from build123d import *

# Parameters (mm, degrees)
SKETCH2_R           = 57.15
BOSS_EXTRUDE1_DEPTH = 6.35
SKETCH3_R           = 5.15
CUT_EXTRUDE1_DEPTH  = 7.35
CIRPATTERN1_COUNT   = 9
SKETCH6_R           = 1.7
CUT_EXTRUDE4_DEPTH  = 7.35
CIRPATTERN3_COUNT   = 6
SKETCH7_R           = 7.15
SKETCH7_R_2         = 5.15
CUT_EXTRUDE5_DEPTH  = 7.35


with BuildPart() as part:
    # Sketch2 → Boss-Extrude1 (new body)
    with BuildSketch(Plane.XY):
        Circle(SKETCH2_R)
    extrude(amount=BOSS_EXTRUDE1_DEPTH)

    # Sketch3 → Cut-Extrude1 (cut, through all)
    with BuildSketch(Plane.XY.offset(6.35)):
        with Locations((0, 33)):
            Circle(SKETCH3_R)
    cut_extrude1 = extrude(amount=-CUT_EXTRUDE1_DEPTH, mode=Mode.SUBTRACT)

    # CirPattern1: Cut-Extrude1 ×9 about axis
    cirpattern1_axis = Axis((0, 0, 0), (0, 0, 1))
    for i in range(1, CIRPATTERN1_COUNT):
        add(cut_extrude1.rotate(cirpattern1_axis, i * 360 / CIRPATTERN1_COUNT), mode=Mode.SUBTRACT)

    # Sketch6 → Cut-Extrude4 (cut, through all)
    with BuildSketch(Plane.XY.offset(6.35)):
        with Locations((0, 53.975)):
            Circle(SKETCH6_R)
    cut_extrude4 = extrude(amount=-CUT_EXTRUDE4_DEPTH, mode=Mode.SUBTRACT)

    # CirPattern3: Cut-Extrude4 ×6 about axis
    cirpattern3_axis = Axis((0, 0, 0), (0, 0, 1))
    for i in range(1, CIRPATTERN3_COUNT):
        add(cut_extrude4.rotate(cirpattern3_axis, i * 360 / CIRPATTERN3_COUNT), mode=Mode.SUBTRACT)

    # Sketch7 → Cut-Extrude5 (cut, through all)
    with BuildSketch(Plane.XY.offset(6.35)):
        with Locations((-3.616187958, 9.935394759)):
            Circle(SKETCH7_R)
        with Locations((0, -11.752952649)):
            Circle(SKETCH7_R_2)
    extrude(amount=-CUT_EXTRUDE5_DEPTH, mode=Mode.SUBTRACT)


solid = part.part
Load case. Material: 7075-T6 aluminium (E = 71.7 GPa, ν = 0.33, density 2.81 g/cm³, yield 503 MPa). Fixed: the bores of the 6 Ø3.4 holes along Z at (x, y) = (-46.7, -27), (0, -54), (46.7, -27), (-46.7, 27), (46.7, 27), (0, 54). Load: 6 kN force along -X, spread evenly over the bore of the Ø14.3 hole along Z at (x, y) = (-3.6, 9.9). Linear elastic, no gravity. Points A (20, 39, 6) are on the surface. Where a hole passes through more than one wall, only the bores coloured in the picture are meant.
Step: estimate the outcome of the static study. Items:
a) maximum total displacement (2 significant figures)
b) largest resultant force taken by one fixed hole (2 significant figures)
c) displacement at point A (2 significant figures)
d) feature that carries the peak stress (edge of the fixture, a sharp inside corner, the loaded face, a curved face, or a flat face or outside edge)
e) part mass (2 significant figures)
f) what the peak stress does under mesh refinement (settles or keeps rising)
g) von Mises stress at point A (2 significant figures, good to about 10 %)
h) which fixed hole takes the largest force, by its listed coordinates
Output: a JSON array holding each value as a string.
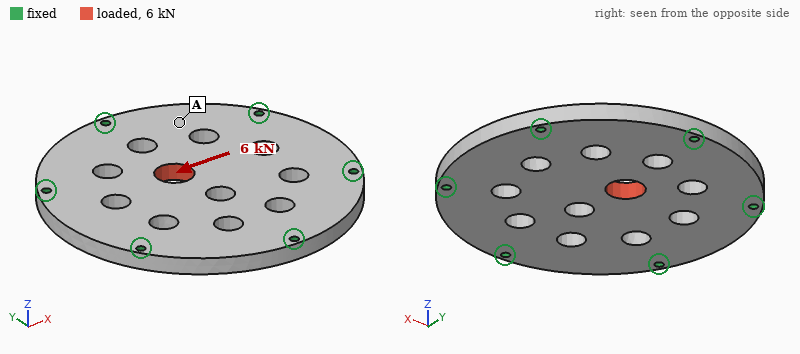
["12 µm", "1.6 kN", "4.1 µm", "edge of the fixture", "160 g", "keeps rising", "5.2 MPa", "(-46.7, 27)"]
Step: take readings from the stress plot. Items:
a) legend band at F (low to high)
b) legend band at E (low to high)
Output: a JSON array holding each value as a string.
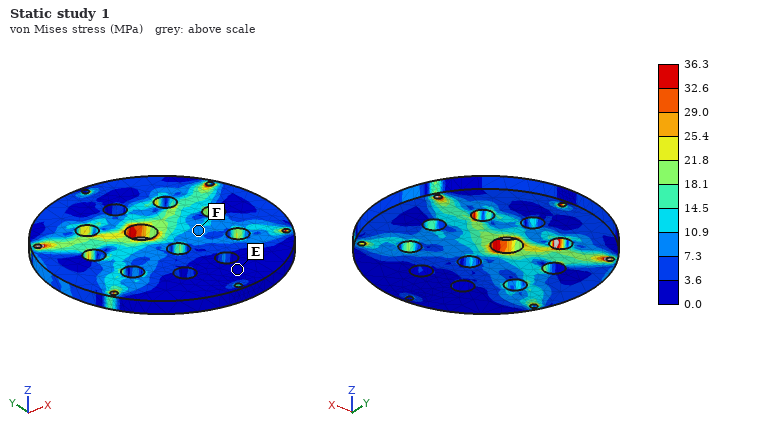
["7.3 to 10.9 MPa", "0.0 to 3.6 MPa"]
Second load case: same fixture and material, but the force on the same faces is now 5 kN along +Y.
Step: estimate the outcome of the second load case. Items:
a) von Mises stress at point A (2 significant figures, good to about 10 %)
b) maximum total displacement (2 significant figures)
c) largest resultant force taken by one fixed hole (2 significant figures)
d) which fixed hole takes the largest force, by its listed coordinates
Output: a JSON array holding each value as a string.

["3.5 MPa", "11 µm", "1.5 kN", "(0, 54)"]
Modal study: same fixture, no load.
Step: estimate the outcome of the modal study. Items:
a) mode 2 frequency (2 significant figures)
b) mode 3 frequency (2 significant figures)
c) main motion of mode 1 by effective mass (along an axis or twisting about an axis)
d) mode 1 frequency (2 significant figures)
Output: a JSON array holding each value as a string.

["7600 Hz", "7700 Hz", "along Z", "3800 Hz"]
